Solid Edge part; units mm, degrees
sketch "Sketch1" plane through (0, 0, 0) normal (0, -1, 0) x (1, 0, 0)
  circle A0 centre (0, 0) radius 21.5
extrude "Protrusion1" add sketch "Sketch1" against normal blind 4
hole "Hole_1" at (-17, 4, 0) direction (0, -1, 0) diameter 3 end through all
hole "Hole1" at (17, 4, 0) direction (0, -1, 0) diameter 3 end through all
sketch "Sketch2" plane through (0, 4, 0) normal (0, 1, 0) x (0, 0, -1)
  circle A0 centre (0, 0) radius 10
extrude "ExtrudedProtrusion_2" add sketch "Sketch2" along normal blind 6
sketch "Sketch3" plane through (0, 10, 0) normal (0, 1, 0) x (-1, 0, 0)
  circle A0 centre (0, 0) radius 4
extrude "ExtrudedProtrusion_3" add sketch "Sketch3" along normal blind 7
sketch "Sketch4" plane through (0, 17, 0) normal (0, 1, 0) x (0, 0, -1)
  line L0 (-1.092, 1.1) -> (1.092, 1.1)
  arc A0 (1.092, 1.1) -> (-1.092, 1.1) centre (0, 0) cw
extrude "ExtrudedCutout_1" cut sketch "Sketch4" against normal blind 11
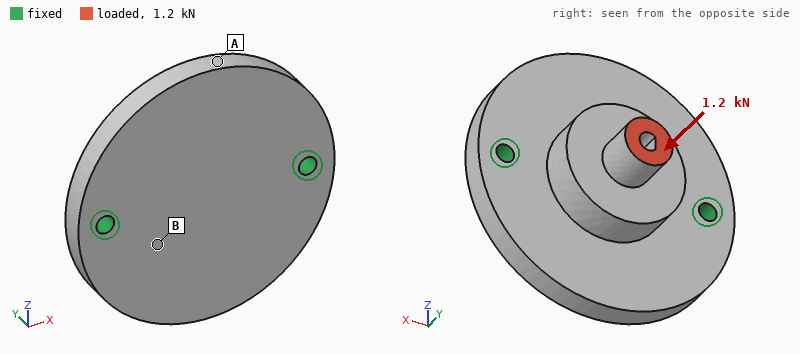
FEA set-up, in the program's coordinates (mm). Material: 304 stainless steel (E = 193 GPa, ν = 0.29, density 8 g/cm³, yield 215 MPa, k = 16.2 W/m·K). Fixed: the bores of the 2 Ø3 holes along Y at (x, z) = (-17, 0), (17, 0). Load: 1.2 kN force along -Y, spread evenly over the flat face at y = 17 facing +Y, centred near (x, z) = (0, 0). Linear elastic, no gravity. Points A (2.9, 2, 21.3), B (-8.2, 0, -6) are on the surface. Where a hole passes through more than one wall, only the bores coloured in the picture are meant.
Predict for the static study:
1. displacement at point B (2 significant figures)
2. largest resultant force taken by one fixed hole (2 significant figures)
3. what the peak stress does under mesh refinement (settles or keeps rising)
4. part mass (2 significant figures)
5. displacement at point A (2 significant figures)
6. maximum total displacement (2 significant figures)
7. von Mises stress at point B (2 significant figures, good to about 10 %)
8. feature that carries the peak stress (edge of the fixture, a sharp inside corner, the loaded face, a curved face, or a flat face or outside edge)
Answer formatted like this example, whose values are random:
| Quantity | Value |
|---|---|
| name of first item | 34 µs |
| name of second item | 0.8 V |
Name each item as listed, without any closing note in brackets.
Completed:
| Quantity | Value |
|---|---|
| displacement at point B | 4.4 µm |
| largest resultant force taken by one fixed hole | 650 N |
| what the peak stress does under mesh refinement | keeps rising |
| part mass | 63 g |
| displacement at point A | 6.1 µm |
| maximum total displacement | 6.4 µm |
| von Mises stress at point B | 19 MPa |
| feature that carries the peak stress | edge of the fixture |
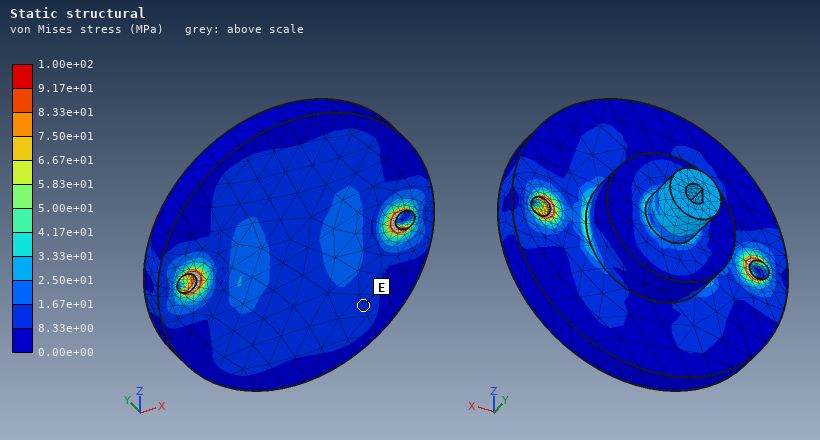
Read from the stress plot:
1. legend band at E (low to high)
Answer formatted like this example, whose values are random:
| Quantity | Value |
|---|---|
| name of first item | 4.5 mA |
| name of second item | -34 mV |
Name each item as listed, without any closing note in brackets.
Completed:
| Quantity | Value |
|---|---|
| legend band at E | 8.33e+00 to 1.67e+01 MPa |
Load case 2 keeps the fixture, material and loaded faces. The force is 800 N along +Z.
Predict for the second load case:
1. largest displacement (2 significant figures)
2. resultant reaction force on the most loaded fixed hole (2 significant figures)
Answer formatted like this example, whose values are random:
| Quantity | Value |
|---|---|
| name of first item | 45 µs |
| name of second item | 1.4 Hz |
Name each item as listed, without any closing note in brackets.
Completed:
| Quantity | Value |
|---|---|
| largest displacement | 36 µm |
| resultant reaction force on the most loaded fixed hole | 400 N |
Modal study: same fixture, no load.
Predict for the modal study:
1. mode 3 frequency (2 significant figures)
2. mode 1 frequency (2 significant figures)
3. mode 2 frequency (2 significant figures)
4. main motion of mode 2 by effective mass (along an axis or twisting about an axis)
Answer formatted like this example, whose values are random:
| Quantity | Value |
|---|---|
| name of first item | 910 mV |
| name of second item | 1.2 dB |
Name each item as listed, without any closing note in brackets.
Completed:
| Quantity | Value |
|---|---|
| mode 3 frequency | 18 kHz |
| mode 1 frequency | 5400 Hz |
| mode 2 frequency | 9900 Hz |
| main motion of mode 2 by effective mass | along Y |
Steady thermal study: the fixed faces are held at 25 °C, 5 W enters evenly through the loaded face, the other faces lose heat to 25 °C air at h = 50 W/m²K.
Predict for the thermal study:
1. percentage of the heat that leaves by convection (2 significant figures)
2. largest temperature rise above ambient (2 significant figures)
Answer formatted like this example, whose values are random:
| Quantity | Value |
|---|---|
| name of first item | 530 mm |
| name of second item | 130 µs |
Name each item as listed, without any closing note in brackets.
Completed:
| Quantity | Value |
|---|---|
| percentage of the heat that leaves by convection | 47 % |
| largest temperature rise above ambient | 74 K |
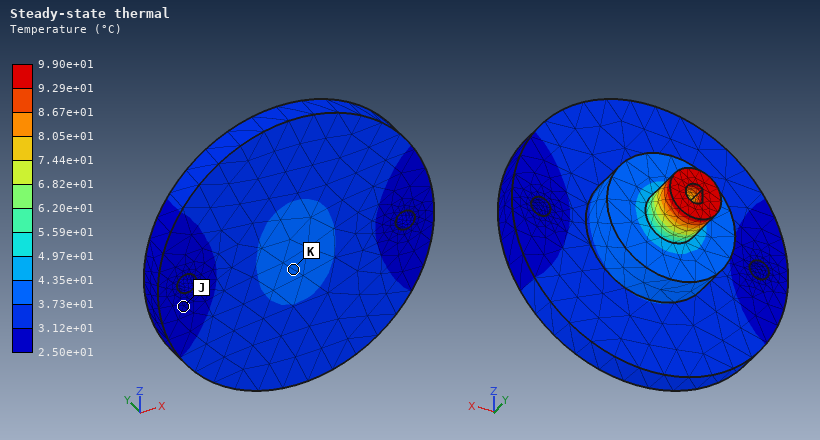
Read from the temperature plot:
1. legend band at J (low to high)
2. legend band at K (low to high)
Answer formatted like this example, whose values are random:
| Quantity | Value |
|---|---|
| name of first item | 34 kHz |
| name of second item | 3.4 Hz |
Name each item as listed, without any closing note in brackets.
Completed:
| Quantity | Value |
|---|---|
| legend band at J | 2.50e+01 to 3.12e+01 °C |
| legend band at K | 3.73e+01 to 4.35e+01 °C |
